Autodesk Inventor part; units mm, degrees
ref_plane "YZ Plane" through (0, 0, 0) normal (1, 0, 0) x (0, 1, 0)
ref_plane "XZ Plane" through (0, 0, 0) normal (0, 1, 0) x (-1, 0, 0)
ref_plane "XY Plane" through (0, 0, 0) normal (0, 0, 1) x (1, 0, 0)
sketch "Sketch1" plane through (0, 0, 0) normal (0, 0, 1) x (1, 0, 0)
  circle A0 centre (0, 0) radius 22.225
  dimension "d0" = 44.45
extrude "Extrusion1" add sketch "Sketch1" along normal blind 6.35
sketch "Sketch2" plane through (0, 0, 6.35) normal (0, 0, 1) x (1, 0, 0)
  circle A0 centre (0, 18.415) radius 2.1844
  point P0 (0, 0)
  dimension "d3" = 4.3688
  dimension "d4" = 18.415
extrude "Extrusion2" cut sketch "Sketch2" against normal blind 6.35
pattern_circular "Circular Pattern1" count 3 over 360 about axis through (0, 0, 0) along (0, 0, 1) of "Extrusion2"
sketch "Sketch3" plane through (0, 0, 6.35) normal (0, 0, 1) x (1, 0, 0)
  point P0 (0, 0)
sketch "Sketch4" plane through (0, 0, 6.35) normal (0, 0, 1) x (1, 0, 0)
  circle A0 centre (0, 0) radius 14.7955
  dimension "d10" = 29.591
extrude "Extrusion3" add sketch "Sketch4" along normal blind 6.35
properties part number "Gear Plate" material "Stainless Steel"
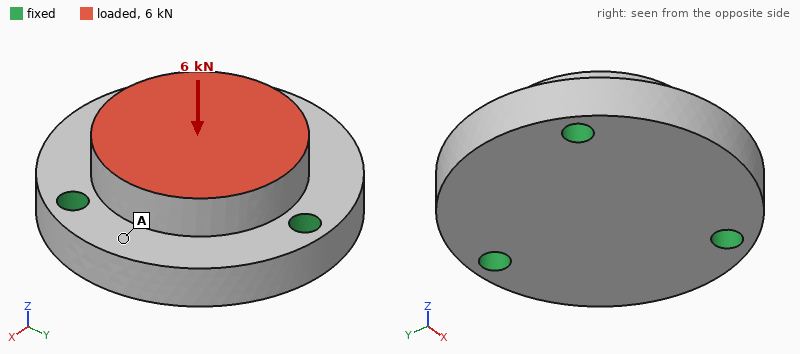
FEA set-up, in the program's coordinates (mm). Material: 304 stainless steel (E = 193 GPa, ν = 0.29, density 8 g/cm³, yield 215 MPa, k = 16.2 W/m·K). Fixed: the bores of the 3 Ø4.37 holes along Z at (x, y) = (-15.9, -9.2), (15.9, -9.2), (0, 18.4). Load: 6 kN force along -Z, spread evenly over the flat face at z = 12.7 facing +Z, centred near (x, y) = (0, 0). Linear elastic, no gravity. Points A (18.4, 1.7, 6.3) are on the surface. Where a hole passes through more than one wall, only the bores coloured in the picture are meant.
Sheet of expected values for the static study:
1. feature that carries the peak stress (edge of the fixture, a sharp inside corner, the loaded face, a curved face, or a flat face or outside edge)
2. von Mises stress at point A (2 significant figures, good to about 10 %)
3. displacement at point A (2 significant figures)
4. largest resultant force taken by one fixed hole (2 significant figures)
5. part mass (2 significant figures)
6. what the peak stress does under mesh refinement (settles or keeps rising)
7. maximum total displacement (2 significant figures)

edge of the fixture
10 MPa
2.3 µm
2.1 kN
110 g
keeps rising
3.7 µm
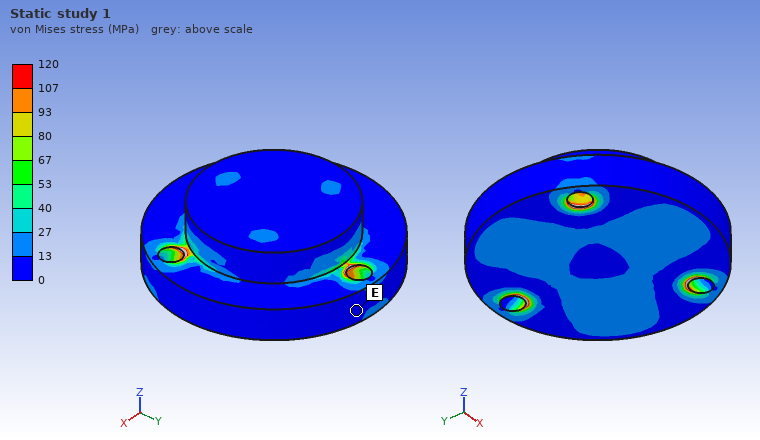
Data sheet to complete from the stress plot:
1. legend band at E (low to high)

0 to 13 MPa
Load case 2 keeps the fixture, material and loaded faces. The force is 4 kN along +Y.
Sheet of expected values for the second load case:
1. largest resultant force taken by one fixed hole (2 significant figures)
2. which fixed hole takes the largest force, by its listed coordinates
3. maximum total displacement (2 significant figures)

2.1 kN
(0, 18.4)
4.1 µm
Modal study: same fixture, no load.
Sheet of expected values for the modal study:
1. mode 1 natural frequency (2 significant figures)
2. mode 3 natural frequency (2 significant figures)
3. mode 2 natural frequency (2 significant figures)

22 kHz
23 kHz
23 kHz
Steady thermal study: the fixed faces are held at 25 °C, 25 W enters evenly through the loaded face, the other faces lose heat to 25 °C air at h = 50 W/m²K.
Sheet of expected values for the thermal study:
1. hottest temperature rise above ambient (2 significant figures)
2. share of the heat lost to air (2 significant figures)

47 K
15 %
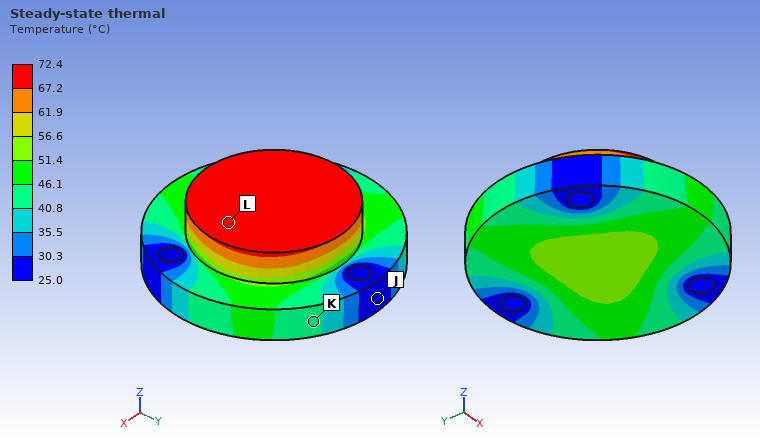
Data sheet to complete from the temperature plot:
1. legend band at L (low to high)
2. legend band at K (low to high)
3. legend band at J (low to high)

67.2 to 72.4 °C
40.8 to 46.1 °C
25.0 to 30.3 °C
